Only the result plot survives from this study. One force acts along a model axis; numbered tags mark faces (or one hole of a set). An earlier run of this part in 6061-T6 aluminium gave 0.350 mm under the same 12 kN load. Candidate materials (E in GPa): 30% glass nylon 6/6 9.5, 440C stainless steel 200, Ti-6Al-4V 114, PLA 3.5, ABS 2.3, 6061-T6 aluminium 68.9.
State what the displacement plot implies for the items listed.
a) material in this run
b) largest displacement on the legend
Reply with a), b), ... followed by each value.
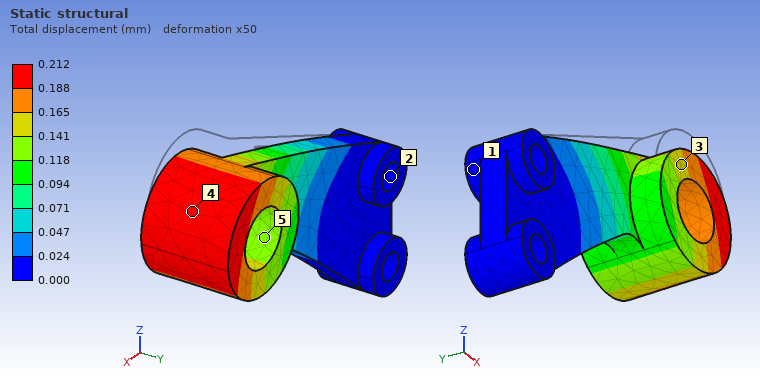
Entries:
a) Ti-6Al-4V
b) 0.212 mm
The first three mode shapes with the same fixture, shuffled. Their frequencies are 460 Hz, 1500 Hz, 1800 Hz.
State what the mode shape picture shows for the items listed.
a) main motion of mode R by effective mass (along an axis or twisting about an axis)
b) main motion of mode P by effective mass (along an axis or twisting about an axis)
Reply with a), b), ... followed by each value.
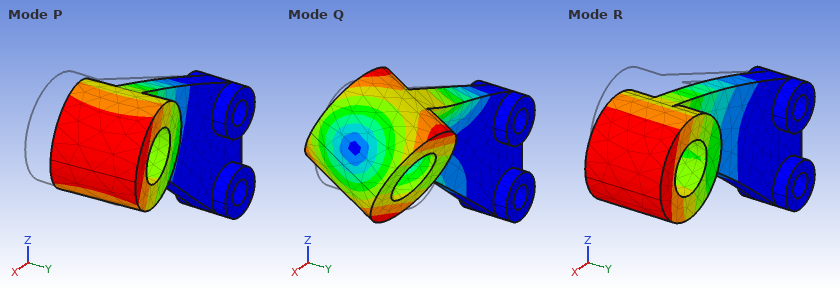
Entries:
a) along Z
b) along Y
